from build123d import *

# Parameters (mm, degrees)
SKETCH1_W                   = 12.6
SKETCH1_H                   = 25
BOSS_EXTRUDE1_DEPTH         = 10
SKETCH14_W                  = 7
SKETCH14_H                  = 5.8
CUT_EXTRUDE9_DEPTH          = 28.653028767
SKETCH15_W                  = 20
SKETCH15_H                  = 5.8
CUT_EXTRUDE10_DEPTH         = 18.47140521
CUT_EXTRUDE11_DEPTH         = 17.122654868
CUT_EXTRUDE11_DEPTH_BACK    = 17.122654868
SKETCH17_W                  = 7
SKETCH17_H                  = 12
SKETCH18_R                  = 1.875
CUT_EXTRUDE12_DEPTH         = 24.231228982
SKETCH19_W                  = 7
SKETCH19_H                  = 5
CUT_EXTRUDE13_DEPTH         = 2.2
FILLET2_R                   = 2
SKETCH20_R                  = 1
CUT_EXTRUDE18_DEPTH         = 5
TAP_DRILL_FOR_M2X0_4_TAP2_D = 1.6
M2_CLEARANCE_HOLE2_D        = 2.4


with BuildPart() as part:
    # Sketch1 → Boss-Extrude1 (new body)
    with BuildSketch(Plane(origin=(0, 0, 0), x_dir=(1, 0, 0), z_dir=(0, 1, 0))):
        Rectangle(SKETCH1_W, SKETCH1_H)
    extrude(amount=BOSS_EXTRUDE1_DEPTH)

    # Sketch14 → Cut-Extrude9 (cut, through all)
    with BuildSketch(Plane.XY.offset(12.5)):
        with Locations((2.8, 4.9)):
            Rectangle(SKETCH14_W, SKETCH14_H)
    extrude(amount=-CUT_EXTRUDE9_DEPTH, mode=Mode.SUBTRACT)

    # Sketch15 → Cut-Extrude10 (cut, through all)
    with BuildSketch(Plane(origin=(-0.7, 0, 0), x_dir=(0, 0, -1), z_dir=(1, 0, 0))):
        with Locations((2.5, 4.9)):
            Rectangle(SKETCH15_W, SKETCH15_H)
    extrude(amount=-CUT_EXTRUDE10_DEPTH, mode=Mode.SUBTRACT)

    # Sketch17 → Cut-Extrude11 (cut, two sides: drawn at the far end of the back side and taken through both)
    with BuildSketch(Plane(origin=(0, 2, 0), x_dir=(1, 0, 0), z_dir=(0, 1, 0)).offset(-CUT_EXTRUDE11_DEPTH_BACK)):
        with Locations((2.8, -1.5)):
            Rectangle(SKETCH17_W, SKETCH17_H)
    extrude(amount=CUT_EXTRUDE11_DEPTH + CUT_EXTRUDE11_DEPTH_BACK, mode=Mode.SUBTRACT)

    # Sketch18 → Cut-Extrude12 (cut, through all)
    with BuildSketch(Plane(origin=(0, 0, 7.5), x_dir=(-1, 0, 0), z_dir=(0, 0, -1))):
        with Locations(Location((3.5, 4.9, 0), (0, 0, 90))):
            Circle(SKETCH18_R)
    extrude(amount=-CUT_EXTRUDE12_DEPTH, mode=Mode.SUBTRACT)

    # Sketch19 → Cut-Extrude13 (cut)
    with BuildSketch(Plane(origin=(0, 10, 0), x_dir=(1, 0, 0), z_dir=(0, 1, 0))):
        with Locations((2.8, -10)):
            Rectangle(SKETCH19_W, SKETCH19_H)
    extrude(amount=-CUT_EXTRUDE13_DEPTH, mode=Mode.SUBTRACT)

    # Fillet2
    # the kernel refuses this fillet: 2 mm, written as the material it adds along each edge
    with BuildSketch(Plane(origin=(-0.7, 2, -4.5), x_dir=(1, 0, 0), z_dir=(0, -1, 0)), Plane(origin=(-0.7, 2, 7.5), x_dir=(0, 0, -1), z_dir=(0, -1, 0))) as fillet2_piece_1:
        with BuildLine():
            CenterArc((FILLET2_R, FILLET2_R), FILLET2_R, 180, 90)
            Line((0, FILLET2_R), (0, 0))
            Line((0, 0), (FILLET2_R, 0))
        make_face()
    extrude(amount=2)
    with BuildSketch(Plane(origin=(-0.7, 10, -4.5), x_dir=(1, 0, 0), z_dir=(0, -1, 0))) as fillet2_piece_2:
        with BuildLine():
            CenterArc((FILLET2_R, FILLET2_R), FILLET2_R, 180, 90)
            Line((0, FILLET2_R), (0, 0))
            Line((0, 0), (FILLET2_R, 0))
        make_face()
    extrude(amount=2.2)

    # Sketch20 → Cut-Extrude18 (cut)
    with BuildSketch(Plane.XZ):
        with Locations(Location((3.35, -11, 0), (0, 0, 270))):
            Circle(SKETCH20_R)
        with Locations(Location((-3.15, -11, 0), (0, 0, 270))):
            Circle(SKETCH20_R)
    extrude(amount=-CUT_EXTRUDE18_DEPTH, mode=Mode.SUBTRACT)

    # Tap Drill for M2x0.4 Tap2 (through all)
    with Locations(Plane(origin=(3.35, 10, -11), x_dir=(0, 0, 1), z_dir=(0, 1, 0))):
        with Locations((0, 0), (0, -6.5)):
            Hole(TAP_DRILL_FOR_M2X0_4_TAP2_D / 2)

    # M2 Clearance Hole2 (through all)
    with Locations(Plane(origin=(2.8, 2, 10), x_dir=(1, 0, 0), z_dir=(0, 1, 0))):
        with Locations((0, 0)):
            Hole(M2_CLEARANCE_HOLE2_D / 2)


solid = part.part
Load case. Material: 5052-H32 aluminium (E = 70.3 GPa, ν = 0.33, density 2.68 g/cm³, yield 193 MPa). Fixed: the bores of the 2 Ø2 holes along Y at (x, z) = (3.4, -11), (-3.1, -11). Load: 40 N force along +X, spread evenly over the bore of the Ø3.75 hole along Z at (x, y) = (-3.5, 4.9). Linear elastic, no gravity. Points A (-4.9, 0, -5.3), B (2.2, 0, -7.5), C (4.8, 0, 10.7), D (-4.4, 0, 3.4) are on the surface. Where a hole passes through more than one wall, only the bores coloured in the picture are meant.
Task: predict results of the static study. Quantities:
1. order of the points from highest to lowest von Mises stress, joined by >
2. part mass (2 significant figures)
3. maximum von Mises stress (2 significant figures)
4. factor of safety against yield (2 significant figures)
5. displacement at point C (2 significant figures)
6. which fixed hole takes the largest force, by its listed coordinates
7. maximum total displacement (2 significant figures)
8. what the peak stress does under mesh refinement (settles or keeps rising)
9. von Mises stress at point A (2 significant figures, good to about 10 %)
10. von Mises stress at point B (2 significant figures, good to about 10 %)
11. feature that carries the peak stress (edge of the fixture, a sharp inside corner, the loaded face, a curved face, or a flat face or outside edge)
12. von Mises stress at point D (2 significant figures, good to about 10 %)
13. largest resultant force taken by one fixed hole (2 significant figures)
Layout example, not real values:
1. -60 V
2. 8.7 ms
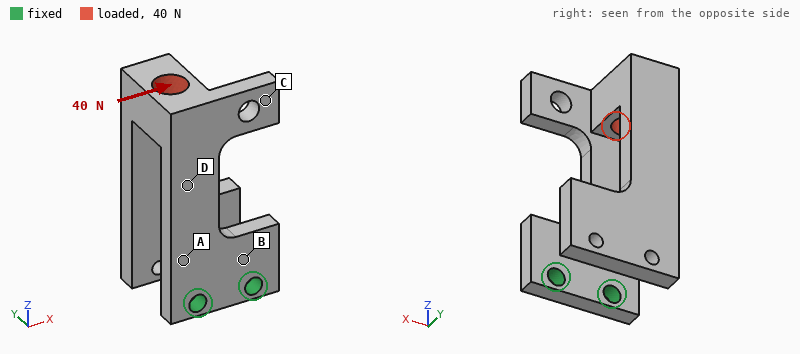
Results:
1. A > D > B > C
2. 2.6 g
3. 100 MPa
4. 1.9
5. 0.066 mm
6. (3.4, -11)
7. 0.11 mm
8. settles
9. 43 MPa
10. 18 MPa
11. a curved face
12. 34 MPa
13. 120 N
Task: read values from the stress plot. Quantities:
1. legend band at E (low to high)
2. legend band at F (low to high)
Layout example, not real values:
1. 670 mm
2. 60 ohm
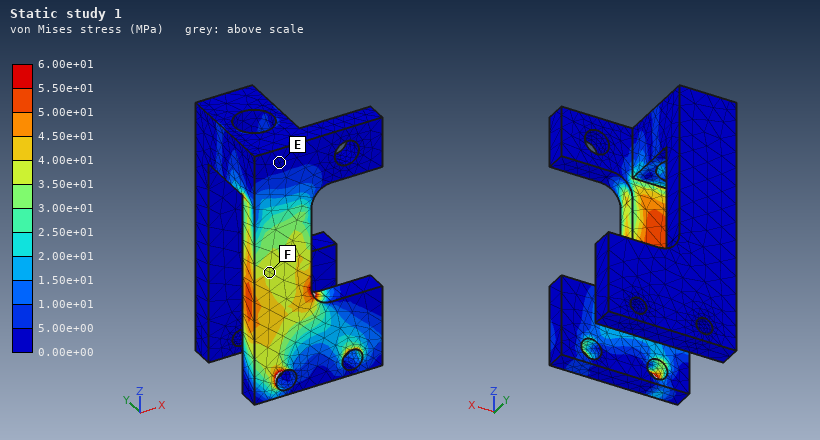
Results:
1. 0.00e+00 to 5.00e+00 MPa
2. 3.50e+01 to 4.00e+01 MPa
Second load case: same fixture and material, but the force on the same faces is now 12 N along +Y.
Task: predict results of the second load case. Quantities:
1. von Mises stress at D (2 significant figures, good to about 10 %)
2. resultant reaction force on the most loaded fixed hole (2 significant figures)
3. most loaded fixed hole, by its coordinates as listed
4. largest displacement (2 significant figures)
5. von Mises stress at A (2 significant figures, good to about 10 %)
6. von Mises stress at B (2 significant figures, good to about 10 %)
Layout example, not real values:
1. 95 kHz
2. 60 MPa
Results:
1. 21 MPa
2. 12 N
3. (-3.1, -11)
4. 0.14 mm
5. 38 MPa
6. 20 MPa
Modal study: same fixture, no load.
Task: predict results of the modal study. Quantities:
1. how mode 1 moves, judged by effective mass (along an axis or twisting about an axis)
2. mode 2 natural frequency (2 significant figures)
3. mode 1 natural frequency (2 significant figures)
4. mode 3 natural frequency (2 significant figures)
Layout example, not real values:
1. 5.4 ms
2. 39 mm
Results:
1. along Z
2. 1900 Hz
3. 1300 Hz
4. 2200 Hz
